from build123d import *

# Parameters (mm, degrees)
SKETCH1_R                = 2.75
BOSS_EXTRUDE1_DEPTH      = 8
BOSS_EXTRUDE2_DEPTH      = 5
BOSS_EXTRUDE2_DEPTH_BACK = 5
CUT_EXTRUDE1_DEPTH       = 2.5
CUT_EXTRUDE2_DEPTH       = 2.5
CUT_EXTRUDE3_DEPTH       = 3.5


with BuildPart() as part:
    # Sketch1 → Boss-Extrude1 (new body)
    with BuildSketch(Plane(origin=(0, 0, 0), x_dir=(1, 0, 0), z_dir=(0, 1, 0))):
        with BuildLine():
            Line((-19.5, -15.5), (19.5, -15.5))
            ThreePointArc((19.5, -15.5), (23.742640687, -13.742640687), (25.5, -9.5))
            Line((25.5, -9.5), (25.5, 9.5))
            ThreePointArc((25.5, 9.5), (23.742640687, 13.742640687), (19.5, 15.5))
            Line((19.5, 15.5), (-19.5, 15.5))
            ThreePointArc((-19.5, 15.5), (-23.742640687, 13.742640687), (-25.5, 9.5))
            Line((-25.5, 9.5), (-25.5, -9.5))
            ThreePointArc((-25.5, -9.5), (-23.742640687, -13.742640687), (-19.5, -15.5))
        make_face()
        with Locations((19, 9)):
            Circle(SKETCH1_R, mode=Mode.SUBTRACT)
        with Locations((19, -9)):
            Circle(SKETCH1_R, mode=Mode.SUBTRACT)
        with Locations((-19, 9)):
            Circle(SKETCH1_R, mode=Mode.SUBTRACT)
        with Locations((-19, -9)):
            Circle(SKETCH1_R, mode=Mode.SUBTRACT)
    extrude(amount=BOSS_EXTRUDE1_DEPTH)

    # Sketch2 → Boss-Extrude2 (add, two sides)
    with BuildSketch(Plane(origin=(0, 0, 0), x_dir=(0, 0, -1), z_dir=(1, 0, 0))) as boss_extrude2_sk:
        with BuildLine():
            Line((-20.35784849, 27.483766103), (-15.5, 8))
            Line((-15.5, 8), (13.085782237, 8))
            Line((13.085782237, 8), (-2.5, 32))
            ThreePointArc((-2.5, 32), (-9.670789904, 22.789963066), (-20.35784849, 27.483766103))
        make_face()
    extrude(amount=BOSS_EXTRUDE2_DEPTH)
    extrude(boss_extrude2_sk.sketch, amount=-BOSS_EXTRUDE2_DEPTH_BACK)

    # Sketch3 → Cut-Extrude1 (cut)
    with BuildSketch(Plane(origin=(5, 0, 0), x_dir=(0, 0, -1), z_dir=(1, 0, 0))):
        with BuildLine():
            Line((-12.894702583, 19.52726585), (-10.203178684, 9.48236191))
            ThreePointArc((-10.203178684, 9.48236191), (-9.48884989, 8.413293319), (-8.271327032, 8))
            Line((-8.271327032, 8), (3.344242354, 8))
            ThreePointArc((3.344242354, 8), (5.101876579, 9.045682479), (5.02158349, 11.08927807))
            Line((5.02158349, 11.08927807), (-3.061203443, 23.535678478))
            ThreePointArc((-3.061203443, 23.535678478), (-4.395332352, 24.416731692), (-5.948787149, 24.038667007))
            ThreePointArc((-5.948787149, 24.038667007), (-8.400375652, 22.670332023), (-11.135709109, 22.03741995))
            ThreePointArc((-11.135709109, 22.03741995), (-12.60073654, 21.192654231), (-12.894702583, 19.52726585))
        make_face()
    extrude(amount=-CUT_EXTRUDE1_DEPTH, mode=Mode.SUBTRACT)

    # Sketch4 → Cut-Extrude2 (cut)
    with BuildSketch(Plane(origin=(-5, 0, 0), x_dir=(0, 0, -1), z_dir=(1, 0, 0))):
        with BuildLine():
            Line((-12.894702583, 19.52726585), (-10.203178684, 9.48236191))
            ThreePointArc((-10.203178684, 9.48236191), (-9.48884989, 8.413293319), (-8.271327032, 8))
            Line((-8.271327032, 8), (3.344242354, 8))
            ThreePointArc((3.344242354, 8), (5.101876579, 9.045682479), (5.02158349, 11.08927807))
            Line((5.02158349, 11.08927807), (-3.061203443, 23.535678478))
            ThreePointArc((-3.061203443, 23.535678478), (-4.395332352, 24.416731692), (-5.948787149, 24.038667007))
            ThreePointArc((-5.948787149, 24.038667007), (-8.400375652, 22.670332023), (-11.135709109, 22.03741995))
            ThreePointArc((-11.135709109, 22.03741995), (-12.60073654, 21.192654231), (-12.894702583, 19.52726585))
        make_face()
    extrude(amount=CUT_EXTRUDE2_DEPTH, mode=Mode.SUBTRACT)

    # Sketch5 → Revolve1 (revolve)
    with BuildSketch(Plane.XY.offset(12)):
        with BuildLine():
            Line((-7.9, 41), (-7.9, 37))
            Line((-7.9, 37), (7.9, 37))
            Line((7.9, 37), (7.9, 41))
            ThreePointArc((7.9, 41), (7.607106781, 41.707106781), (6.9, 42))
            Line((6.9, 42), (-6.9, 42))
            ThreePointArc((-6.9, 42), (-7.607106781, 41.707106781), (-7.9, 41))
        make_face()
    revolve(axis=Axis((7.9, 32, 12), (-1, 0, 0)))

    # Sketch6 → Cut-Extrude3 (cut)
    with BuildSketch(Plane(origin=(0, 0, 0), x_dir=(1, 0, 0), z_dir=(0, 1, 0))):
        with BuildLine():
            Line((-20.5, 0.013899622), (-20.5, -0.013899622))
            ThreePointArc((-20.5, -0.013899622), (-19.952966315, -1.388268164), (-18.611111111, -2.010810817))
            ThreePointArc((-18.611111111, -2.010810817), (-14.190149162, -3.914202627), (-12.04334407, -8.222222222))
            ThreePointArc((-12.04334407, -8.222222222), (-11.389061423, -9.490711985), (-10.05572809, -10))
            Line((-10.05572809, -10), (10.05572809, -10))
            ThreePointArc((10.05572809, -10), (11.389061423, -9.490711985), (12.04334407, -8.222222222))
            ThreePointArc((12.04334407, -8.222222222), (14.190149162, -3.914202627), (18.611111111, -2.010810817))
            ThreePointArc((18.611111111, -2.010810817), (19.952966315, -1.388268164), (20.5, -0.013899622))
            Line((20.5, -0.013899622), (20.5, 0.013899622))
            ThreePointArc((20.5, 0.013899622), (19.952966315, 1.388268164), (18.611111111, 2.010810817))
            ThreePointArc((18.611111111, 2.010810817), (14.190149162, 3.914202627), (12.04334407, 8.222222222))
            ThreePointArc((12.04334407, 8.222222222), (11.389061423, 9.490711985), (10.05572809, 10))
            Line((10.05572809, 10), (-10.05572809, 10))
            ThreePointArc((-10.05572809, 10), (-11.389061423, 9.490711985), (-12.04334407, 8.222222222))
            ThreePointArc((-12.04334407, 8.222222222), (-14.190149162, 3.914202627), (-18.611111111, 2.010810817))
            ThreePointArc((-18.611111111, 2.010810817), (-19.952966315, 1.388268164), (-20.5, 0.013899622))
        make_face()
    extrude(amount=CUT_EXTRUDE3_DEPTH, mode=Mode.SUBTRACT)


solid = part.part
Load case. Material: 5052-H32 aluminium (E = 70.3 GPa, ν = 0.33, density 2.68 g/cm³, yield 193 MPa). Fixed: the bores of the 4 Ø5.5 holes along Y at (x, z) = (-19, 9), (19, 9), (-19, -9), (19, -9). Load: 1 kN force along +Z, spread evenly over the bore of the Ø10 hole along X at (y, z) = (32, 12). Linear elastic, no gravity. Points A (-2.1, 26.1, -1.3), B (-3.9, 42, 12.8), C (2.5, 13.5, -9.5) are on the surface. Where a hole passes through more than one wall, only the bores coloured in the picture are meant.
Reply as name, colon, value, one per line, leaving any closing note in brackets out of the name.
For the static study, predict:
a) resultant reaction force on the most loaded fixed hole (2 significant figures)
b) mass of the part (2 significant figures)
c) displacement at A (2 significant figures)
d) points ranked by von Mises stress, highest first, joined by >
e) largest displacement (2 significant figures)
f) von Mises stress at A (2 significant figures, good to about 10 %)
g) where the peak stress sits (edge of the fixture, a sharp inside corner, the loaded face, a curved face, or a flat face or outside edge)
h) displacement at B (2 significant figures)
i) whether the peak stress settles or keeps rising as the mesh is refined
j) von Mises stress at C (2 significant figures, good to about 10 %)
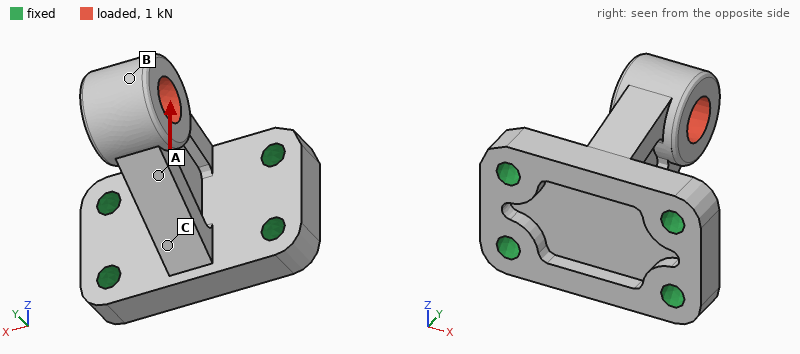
resultant reaction force on the most loaded fixed hole: 700 N
mass of the part: 44 g
displacement at A: 30 µm
points ranked by von Mises stress, highest first, joined by >: C > A > B
largest displacement: 59 µm
von Mises stress at A: 17 MPa
where the peak stress sits: edge of the fixture
displacement at B: 58 µm
whether the peak stress settles or keeps rising as the mesh is refined: keeps rising
von Mises stress at C: 28 MPa
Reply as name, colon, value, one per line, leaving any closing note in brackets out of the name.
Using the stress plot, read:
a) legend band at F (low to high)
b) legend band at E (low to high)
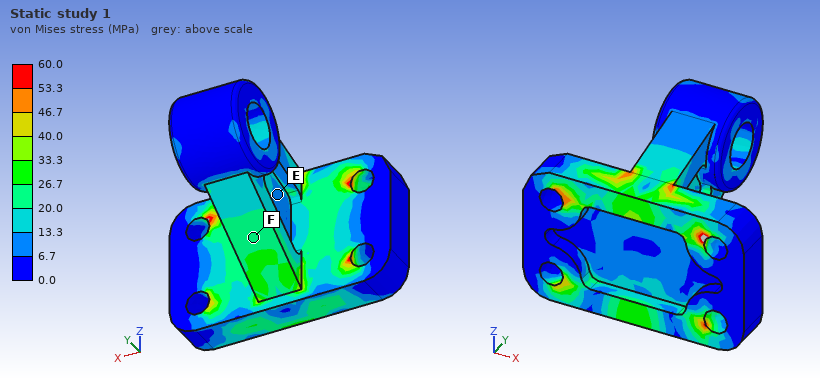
legend band at F: 20.0 to 26.7 MPa
legend band at E: 6.7 to 13.3 MPa
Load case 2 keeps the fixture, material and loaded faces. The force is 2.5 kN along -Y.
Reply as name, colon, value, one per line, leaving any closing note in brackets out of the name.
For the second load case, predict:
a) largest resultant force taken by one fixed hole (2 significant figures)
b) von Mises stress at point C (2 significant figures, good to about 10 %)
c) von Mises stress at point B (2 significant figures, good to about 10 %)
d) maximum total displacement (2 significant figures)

largest resultant force taken by one fixed hole: 1.3 kN
von Mises stress at point C: 12 MPa
von Mises stress at point B: 11 MPa
maximum total displacement: 63 µm
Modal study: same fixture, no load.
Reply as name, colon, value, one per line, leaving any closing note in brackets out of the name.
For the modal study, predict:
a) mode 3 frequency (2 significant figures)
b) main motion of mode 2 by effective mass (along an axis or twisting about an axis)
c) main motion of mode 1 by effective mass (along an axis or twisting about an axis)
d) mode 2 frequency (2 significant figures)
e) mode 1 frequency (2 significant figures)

mode 3 frequency: 12 kHz
main motion of mode 2 by effective mass: along Z
main motion of mode 1 by effective mass: along X
mode 2 frequency: 6500 Hz
mode 1 frequency: 4200 Hz
